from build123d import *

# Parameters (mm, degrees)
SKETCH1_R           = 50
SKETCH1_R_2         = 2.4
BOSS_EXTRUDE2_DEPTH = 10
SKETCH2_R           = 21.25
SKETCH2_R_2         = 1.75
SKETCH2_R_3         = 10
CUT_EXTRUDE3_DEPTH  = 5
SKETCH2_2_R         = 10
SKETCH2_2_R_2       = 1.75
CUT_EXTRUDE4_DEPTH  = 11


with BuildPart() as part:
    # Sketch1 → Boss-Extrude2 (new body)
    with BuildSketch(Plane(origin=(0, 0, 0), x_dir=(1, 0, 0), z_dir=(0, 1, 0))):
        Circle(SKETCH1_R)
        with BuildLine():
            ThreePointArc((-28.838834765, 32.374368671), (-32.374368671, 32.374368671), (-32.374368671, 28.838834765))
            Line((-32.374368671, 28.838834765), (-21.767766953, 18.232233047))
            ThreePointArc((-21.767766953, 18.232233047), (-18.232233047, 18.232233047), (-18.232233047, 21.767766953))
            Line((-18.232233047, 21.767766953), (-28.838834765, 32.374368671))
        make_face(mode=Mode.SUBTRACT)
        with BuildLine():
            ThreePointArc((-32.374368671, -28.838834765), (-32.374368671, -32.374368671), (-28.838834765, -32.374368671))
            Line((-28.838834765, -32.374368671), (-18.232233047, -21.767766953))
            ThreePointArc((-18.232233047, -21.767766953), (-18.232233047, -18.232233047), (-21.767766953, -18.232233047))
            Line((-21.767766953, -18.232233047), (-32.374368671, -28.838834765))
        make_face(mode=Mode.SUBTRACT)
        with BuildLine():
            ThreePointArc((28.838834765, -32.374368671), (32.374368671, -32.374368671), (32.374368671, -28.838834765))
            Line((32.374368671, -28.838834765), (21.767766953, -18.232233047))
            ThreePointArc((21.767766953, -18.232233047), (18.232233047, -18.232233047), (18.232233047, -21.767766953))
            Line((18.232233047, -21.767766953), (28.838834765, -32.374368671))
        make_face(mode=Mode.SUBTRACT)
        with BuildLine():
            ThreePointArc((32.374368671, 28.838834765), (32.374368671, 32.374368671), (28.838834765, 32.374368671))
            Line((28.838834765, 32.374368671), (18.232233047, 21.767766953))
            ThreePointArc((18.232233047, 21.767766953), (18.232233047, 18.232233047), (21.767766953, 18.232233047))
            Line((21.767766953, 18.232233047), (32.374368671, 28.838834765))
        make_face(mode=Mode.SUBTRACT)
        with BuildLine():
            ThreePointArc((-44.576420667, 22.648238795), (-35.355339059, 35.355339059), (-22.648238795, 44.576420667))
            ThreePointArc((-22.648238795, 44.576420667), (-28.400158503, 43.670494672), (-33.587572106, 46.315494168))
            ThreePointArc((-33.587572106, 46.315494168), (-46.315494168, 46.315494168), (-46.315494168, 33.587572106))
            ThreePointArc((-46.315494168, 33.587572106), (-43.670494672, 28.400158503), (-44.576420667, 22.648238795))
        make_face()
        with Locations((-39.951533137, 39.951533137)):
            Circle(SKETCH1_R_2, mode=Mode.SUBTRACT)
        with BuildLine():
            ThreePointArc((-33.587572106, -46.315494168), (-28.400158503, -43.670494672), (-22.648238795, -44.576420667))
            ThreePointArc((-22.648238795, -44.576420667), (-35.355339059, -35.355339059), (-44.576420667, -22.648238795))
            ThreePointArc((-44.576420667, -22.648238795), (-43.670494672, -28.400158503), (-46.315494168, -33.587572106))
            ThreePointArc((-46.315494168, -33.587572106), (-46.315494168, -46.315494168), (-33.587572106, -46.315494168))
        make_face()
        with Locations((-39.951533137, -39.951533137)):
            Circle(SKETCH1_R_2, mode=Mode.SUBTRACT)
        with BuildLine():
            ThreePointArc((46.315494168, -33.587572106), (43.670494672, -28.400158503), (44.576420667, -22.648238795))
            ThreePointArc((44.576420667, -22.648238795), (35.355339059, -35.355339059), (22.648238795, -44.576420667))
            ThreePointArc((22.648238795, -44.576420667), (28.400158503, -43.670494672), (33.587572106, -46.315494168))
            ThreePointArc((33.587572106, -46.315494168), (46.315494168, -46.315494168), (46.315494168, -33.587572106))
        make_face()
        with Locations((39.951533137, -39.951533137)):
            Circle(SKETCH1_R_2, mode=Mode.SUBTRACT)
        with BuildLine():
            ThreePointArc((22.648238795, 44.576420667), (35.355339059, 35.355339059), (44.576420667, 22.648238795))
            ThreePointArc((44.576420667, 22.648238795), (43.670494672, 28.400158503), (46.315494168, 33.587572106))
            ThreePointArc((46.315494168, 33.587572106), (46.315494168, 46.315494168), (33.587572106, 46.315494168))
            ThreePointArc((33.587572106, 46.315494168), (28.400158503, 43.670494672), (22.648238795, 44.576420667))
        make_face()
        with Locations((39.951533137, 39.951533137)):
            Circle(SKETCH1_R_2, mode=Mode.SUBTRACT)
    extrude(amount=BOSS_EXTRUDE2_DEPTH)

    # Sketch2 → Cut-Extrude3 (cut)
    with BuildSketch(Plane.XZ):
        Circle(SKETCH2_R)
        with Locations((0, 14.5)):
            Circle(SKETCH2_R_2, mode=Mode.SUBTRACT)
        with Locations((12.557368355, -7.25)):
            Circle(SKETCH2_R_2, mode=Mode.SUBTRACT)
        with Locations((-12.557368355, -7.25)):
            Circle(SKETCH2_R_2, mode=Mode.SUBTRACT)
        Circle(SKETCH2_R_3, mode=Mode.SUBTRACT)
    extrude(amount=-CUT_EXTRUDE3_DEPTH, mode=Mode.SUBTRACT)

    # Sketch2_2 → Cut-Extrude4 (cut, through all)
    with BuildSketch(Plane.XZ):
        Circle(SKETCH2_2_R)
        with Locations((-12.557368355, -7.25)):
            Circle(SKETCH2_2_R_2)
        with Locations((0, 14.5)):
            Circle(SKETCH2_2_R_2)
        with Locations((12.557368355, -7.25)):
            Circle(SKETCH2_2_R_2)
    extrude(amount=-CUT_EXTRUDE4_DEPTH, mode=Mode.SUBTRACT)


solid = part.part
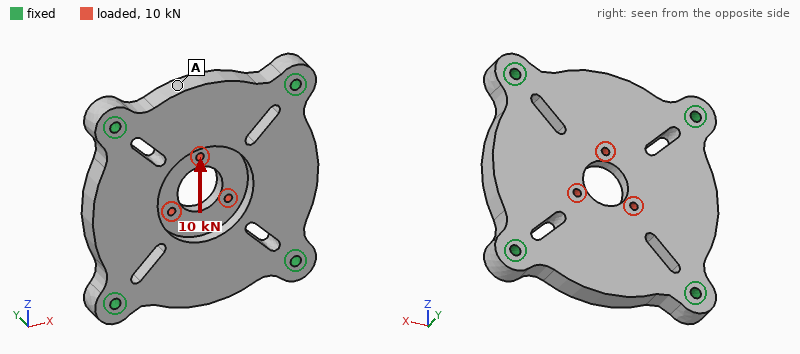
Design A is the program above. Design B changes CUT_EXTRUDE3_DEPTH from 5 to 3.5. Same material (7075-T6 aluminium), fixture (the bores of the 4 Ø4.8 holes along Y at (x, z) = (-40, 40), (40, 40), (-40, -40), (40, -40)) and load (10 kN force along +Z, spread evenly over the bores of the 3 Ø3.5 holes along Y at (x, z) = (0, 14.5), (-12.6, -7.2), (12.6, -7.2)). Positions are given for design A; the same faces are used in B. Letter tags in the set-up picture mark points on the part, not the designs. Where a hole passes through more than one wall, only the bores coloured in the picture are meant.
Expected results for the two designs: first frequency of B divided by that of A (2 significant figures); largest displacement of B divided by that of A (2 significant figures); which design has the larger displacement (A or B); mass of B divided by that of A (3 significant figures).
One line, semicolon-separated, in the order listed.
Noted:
0.97; 0.86; A; 1.02
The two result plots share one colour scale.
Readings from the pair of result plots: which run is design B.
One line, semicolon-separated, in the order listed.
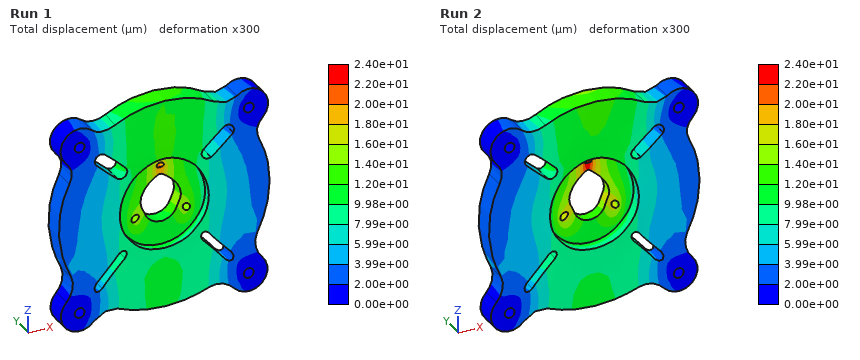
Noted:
Run 1
